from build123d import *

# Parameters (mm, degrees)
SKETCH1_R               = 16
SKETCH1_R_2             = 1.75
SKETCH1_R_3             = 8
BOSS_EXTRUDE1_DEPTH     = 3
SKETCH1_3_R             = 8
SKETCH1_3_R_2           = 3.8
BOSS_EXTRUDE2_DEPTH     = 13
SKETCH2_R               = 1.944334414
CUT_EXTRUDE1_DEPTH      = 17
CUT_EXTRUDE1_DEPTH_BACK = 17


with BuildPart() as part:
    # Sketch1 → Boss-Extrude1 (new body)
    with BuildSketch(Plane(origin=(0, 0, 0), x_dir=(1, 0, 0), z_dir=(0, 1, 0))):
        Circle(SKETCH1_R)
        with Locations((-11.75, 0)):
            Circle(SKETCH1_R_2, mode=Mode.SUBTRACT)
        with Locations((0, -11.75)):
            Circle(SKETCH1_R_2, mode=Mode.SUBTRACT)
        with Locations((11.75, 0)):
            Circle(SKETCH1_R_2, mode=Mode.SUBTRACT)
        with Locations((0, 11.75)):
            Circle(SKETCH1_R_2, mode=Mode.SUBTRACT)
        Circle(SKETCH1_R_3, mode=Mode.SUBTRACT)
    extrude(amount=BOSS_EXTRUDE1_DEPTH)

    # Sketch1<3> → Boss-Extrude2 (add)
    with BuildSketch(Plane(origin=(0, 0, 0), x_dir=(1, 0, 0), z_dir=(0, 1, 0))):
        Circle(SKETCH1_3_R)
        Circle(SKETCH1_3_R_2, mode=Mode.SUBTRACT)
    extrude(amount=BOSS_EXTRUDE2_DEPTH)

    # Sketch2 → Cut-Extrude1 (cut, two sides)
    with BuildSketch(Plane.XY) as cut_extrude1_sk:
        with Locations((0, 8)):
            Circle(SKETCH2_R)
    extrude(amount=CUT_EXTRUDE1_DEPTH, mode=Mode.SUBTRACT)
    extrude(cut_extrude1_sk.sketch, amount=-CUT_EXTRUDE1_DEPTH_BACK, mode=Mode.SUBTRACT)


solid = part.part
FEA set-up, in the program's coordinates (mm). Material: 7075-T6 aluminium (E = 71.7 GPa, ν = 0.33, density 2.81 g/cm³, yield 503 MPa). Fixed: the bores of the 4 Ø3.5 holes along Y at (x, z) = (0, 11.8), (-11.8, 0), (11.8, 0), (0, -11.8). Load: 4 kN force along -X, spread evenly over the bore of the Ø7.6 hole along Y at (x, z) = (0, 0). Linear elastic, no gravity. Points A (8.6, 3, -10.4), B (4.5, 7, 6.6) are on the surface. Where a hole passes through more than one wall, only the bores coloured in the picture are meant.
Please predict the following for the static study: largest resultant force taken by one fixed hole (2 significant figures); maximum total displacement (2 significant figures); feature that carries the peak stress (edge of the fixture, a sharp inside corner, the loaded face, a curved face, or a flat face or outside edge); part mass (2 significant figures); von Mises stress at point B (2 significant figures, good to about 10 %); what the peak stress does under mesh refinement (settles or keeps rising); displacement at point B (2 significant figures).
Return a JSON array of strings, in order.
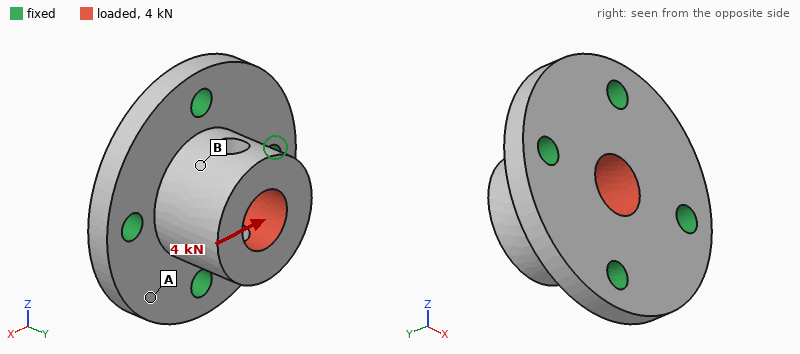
["1.6 kN", "26 µm", "edge of the fixture", "10 g", "36 MPa", "keeps rising", "12 µm"]
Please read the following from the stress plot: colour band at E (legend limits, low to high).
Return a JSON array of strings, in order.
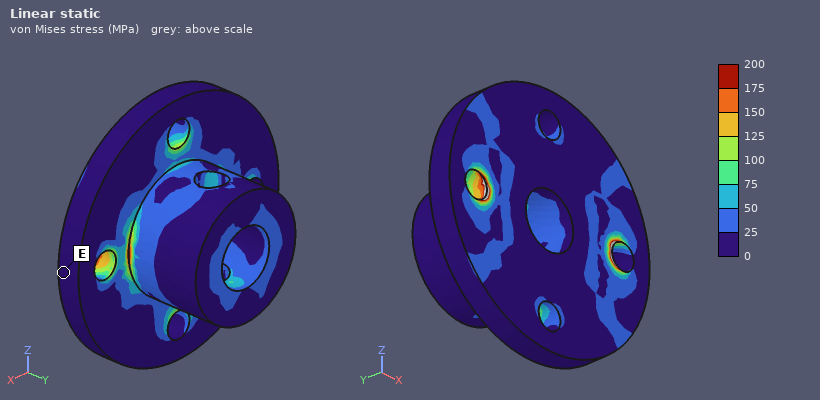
["0 to 25 MPa"]
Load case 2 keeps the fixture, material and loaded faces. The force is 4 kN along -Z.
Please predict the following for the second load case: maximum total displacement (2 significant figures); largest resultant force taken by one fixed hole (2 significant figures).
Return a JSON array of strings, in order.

["25 µm", "1.6 kN"]
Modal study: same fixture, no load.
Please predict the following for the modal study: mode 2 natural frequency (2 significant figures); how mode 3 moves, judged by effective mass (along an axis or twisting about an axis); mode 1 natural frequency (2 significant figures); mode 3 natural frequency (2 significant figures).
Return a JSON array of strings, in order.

["31 kHz", "along Y", "30 kHz", "37 kHz"]
